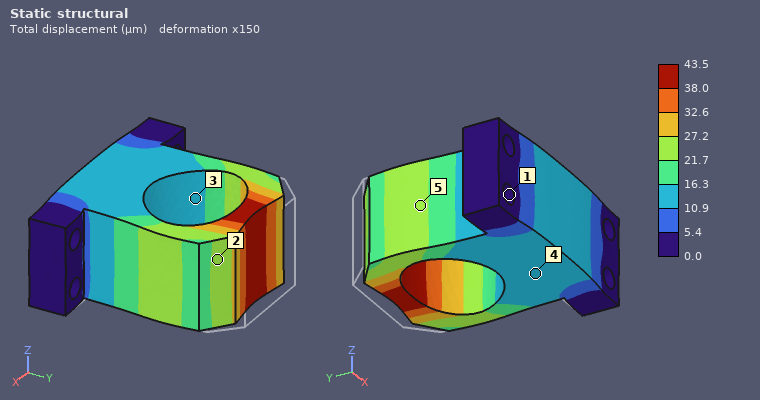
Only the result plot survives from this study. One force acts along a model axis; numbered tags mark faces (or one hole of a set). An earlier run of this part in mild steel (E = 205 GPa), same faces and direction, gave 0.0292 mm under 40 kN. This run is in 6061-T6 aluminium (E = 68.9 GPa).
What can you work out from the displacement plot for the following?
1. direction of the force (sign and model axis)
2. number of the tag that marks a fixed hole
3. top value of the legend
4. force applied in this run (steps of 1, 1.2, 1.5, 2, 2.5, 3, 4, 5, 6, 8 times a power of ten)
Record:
-Y
1
43.5 µm
20 kN
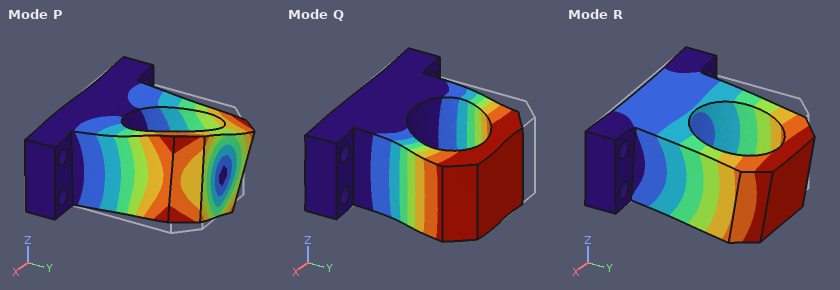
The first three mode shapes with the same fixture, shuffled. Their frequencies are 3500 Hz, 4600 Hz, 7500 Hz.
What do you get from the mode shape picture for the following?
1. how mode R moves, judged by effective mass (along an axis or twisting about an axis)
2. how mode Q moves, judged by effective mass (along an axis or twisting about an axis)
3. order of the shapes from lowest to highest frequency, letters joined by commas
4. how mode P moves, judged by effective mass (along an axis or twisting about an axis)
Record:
along Z
along X
R, Q, P
twisting about Y
